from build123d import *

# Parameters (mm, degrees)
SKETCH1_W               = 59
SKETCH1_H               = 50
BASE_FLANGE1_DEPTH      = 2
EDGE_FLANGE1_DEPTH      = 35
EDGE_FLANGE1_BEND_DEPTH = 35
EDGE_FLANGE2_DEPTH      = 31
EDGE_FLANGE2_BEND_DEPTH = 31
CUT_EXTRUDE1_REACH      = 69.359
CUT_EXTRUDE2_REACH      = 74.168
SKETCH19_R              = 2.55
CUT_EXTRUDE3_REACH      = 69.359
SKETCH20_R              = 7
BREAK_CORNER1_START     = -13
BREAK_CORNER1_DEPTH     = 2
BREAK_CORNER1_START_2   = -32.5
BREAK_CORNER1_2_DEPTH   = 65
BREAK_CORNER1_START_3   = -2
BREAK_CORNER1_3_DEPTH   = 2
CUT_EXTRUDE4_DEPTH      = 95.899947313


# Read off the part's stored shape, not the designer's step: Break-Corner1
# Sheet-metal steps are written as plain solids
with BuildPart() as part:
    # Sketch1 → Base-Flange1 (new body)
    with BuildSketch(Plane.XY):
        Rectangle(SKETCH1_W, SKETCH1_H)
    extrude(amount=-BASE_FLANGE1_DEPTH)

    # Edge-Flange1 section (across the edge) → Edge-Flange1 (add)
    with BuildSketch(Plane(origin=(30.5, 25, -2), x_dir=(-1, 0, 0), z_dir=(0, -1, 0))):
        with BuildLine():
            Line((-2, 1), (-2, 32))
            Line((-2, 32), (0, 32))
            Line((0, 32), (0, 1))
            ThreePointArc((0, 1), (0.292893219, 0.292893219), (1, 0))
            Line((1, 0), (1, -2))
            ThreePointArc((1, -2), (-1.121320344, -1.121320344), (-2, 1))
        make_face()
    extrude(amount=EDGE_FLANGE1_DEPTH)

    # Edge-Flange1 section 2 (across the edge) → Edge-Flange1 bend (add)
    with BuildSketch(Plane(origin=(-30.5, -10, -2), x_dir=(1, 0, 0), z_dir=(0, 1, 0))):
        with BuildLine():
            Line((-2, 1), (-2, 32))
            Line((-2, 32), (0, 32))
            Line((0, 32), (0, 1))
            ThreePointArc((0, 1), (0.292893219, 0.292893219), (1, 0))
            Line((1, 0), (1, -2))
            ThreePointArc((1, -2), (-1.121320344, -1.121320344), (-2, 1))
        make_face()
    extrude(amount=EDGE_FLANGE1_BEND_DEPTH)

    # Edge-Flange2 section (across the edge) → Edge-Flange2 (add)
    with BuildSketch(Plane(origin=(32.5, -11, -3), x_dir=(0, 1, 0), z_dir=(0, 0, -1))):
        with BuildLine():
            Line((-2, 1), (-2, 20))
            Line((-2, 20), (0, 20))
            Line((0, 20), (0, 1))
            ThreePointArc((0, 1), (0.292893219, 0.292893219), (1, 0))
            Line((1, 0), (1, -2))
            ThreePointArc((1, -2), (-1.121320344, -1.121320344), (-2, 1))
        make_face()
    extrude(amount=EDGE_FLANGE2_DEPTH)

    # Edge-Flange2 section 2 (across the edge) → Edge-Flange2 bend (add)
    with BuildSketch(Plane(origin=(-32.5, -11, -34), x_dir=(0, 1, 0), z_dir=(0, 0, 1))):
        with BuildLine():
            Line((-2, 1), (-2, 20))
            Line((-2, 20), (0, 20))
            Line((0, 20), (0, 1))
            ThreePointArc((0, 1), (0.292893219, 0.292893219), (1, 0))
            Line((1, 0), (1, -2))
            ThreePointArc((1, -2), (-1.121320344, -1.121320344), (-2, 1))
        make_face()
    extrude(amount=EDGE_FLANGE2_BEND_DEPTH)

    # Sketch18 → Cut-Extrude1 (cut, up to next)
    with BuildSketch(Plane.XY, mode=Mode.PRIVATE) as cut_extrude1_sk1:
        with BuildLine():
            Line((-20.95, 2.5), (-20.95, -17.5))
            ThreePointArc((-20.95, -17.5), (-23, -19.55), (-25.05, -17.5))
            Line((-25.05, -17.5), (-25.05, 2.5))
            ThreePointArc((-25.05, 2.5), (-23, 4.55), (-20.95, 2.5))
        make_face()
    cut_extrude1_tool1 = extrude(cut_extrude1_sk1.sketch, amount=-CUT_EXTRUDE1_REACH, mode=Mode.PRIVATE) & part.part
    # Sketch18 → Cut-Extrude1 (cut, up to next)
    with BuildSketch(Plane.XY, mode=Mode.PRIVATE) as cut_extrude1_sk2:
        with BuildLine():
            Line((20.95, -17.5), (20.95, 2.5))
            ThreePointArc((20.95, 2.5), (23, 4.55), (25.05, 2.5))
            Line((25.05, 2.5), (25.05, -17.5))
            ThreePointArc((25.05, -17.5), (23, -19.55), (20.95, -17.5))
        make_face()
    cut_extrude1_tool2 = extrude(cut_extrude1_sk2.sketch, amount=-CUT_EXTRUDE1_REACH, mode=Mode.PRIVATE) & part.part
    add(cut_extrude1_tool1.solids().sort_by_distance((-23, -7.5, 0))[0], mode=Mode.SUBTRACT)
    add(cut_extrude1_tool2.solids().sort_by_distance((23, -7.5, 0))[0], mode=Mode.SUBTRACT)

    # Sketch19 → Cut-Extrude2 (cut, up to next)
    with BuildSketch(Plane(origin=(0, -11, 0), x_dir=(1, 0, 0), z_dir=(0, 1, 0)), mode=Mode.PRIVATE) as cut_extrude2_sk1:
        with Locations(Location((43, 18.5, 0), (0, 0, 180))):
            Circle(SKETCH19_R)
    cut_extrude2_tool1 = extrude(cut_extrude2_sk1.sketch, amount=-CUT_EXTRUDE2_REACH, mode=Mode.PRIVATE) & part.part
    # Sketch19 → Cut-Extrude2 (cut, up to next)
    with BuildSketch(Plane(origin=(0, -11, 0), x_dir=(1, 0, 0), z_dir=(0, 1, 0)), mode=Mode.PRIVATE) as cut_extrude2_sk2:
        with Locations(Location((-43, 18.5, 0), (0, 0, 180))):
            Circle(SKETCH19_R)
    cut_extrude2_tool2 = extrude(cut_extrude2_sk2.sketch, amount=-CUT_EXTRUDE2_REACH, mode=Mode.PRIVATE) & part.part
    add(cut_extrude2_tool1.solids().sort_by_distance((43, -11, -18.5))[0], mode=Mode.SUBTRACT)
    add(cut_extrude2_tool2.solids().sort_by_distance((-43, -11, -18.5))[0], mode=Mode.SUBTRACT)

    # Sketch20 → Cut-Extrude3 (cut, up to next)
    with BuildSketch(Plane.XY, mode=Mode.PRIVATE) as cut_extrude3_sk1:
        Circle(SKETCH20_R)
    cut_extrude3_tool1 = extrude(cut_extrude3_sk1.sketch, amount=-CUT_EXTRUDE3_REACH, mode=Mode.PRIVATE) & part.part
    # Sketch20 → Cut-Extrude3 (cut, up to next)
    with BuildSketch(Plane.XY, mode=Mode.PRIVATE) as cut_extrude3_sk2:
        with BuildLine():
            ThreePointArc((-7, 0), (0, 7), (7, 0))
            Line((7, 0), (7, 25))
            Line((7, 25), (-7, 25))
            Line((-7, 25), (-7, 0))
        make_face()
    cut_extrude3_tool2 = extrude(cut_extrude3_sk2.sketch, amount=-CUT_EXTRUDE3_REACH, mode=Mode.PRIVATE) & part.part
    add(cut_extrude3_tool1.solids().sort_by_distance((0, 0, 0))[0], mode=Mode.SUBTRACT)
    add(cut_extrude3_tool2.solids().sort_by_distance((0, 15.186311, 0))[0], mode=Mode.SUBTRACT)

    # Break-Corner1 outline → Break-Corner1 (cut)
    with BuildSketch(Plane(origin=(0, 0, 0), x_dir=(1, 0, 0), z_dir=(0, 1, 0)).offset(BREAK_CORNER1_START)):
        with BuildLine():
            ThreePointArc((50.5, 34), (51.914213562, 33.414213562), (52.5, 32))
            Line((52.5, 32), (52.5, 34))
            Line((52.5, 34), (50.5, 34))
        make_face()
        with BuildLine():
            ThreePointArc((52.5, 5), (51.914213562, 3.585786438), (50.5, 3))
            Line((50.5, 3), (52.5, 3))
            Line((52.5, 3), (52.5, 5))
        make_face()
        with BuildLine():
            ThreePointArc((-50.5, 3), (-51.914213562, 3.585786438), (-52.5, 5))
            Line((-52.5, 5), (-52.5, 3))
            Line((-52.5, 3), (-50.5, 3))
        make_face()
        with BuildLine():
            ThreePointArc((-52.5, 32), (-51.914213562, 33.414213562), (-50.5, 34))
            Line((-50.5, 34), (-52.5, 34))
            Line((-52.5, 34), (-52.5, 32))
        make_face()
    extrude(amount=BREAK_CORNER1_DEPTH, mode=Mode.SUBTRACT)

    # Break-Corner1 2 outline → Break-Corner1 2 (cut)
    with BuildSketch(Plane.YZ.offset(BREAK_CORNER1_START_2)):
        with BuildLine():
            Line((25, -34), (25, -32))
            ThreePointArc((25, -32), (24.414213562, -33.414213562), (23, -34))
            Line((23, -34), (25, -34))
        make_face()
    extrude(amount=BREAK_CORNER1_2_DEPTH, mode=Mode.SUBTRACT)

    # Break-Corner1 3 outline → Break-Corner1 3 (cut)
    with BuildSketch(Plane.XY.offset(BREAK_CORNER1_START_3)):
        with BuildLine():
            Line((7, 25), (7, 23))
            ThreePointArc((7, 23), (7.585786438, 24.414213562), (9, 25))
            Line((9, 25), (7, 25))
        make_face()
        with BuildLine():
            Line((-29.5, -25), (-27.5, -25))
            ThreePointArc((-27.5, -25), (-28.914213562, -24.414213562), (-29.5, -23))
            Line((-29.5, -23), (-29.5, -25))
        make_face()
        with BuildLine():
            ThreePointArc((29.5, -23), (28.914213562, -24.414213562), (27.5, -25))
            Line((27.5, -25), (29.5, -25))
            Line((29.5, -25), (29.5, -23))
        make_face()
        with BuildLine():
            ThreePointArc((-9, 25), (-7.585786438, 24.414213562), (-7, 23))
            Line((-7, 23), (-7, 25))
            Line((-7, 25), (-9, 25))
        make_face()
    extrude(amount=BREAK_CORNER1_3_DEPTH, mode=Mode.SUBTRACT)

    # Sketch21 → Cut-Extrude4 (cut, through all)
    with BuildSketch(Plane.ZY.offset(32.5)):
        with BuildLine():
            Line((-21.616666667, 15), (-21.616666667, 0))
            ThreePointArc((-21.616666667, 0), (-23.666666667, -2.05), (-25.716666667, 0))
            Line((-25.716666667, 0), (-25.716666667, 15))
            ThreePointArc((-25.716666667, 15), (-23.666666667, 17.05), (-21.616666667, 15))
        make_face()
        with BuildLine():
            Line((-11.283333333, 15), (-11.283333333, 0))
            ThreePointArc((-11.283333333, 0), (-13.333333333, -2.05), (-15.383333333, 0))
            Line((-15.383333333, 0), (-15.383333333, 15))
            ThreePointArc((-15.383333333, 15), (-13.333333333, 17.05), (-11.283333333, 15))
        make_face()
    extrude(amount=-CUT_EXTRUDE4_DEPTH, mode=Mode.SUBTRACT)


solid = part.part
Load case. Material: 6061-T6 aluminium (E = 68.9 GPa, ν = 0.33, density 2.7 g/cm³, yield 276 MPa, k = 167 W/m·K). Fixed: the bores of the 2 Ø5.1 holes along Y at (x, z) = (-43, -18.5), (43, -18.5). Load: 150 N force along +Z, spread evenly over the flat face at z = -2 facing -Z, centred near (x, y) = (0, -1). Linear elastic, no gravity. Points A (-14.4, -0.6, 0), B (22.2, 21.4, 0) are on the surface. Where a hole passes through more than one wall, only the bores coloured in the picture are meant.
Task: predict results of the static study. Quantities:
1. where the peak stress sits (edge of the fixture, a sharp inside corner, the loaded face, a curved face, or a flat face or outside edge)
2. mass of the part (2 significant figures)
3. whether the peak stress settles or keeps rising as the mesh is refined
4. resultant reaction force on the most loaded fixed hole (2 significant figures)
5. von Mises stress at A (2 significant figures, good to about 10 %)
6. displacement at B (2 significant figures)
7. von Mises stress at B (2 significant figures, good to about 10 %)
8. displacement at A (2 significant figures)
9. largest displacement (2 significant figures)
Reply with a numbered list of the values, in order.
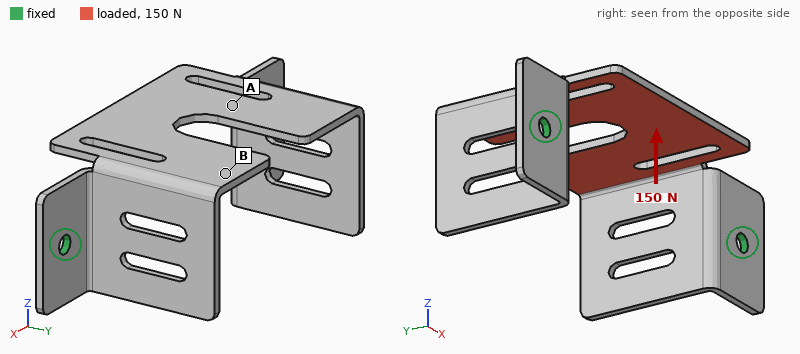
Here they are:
1. a sharp inside corner
2. 31 g
3. keeps rising
4. 88 N
5. 18 MPa
6. 0.17 mm
7. 7.2 MPa
8. 0.18 mm
9. 0.29 mm
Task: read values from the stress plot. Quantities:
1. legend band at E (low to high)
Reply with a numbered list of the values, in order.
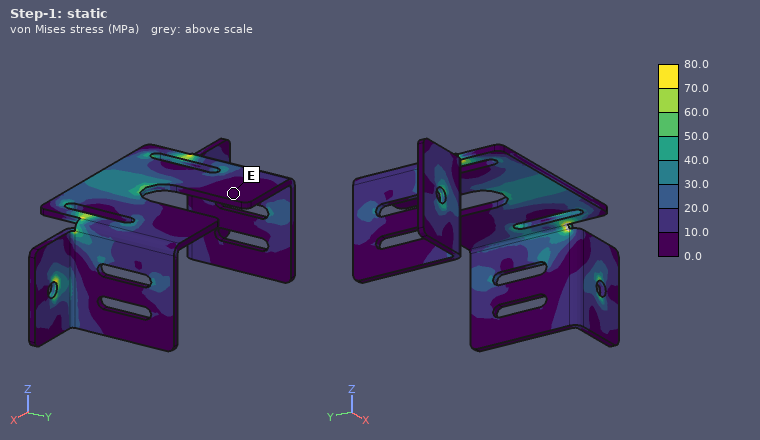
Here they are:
1. 0.0 to 10.0 MPa
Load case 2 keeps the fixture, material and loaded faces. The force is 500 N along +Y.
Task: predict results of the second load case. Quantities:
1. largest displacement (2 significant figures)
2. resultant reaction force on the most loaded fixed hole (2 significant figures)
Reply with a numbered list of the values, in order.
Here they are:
1. 0.67 mm
2. 270 N
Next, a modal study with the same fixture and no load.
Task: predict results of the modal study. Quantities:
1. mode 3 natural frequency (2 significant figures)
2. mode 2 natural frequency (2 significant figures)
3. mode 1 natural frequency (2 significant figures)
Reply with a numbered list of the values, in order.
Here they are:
1. 1300 Hz
2. 1100 Hz
3. 910 Hz
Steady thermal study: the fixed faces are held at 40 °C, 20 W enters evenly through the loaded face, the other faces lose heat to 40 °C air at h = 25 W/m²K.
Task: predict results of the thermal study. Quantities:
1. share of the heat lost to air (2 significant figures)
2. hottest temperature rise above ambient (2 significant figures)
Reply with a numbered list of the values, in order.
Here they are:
1. 29 %
2. 50 K
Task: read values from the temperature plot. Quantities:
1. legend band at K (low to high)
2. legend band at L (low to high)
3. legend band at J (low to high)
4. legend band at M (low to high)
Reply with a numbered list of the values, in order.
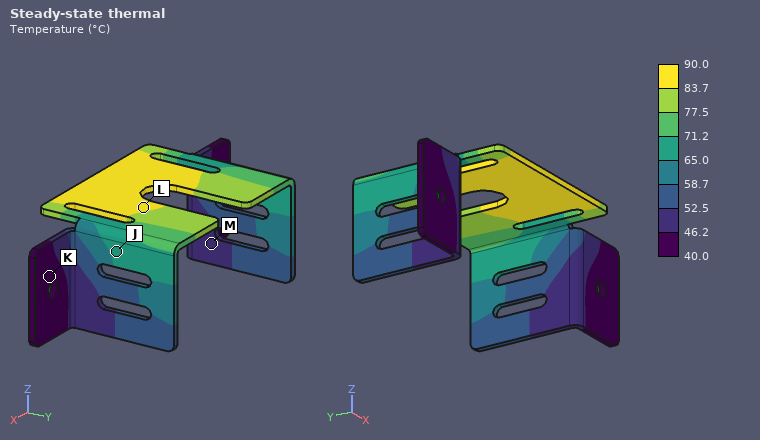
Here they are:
1. 40.0 to 46.2 °C
2. 83.7 to 90.0 °C
3. 65.0 to 71.2 °C
4. 46.2 to 52.5 °C
